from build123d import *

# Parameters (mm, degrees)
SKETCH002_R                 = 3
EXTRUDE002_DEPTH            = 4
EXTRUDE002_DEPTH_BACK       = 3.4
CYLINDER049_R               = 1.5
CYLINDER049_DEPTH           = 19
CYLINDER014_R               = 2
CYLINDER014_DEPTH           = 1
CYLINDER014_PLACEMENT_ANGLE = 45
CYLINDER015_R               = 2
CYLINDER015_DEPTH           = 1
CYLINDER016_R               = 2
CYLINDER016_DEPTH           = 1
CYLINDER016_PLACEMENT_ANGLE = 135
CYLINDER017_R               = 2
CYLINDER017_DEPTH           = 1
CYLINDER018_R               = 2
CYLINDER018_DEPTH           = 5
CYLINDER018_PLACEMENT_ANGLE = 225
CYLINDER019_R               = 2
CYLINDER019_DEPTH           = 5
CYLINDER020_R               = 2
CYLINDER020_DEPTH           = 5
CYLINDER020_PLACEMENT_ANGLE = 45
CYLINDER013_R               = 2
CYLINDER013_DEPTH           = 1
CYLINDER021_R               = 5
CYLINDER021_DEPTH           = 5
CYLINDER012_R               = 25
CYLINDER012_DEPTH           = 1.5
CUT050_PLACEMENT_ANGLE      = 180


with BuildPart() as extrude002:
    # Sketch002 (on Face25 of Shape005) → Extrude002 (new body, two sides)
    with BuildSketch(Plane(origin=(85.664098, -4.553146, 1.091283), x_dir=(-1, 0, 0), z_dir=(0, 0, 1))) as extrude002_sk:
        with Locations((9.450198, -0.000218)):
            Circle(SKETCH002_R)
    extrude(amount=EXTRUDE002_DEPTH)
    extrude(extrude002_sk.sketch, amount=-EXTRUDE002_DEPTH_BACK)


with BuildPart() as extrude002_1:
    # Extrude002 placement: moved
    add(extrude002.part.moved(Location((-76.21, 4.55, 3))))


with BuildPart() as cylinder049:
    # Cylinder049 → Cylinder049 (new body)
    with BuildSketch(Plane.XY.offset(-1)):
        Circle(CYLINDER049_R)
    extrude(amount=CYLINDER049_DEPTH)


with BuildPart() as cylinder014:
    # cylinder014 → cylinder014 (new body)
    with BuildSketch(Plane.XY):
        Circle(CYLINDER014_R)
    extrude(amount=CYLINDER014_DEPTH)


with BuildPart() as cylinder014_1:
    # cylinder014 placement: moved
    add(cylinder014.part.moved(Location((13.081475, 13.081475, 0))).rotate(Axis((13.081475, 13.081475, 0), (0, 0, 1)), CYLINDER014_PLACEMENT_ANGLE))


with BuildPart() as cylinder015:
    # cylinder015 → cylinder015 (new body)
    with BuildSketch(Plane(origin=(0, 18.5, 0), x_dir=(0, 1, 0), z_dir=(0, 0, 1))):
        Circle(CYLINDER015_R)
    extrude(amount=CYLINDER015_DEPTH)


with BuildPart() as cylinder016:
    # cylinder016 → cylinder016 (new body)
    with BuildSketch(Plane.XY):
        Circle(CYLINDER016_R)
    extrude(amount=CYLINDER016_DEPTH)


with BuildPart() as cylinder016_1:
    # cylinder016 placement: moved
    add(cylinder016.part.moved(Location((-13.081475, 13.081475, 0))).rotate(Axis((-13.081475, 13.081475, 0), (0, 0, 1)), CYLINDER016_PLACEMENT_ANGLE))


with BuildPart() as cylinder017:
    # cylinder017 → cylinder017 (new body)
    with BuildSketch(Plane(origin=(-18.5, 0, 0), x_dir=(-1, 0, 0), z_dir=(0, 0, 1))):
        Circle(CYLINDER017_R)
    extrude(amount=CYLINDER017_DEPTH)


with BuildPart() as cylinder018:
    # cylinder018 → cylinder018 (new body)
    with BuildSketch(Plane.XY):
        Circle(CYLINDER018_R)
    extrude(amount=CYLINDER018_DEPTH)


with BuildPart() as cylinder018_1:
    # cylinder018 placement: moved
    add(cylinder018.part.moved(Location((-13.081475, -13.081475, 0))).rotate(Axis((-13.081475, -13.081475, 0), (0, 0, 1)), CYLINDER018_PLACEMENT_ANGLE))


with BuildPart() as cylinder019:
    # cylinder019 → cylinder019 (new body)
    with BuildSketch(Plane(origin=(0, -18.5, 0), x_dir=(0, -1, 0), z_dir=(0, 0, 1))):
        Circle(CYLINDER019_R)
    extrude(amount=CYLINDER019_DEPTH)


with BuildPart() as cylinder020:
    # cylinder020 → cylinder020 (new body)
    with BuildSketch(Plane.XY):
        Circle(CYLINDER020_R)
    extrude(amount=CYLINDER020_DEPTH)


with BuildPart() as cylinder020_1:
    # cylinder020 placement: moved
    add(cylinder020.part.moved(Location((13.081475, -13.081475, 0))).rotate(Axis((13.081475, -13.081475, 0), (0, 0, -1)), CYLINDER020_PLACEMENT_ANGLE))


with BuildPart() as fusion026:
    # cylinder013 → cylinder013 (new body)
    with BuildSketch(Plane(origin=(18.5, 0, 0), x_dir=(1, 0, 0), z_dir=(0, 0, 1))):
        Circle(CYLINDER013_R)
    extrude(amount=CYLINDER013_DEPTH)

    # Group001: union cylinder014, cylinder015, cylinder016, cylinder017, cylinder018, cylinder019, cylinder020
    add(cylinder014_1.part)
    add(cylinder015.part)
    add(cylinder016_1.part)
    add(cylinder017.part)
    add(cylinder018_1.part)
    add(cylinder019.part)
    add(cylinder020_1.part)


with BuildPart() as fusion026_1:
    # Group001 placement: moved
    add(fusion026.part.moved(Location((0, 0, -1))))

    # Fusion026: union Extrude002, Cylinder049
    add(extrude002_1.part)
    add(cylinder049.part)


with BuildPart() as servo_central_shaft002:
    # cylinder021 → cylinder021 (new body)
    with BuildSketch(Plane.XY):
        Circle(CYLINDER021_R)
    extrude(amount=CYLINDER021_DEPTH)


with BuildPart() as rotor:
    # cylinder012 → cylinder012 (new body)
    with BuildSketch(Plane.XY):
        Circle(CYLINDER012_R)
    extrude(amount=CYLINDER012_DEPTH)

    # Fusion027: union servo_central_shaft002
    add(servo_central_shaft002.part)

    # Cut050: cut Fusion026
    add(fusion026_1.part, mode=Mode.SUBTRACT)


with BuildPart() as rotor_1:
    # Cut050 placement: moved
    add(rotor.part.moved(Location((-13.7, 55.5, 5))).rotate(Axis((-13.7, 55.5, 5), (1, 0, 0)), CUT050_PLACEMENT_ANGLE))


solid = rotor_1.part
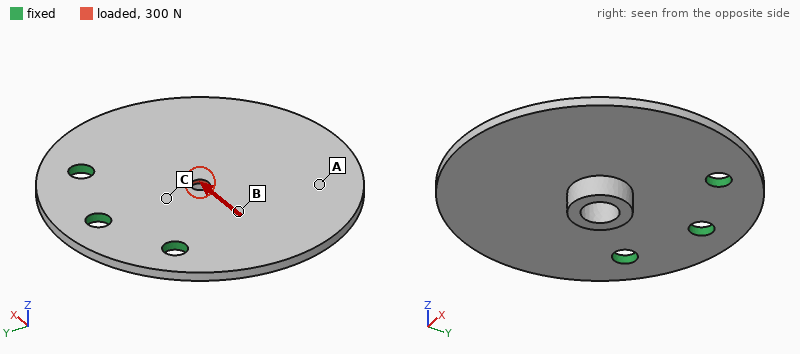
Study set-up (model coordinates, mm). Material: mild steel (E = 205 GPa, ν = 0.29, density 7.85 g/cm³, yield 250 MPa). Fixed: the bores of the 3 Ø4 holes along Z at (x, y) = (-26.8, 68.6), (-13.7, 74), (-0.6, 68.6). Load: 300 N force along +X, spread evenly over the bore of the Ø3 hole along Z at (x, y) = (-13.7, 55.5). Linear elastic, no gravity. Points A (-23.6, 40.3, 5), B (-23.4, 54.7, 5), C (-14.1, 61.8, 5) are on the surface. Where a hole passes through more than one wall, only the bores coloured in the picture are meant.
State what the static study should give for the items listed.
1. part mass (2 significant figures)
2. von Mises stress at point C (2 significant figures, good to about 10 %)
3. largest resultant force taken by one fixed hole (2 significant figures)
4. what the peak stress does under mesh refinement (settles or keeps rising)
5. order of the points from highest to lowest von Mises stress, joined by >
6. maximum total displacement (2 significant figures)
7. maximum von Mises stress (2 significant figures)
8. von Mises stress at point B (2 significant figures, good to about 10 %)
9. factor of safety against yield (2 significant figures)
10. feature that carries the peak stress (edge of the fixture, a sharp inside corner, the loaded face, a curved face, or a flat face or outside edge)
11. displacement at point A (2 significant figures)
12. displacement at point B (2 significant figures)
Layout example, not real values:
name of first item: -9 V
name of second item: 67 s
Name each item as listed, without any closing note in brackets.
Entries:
part mass: 24 g
von Mises stress at point C: 15 MPa
largest resultant force taken by one fixed hole: 190 N
what the peak stress does under mesh refinement: settles
order of the points from highest to lowest von Mises stress, joined by >: C > B > A
maximum total displacement: 3.4 µm
maximum von Mises stress: 81 MPa
von Mises stress at point B: 8.1 MPa
factor of safety against yield: 3.1
feature that carries the peak stress: the loaded face
displacement at point A: 2.4 µm
displacement at point B: 1.7 µm
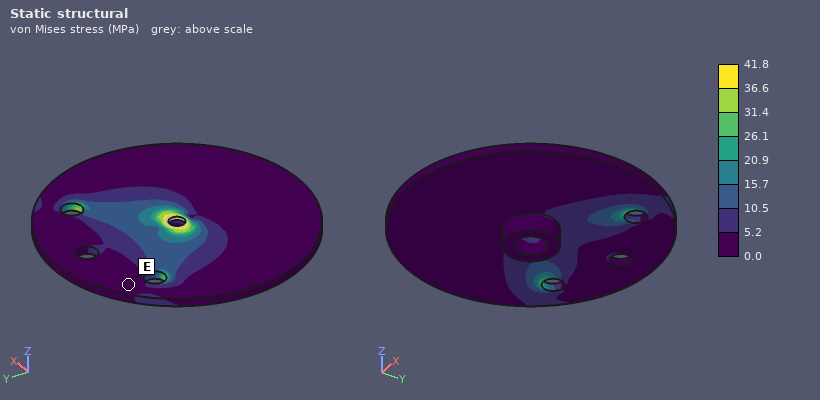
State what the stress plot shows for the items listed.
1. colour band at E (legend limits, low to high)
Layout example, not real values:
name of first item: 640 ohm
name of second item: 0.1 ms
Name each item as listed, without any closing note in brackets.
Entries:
colour band at E: 0.0 to 5.2 MPa
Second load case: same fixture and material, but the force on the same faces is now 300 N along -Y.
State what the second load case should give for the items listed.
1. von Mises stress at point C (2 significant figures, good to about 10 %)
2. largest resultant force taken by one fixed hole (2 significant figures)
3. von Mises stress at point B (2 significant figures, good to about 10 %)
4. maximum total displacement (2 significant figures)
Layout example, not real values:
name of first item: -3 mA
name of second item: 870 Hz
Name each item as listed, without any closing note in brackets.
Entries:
von Mises stress at point C: 20 MPa
largest resultant force taken by one fixed hole: 110 N
von Mises stress at point B: 5.4 MPa
maximum total displacement: 16 µm
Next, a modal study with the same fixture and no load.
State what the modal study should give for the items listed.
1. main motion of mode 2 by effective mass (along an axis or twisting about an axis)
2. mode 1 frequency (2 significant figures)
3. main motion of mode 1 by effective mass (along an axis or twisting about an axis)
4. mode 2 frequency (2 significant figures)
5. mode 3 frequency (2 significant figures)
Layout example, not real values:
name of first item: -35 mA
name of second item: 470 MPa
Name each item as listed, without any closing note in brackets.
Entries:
main motion of mode 2 by effective mass: twisting about Y
mode 1 frequency: 1100 Hz
main motion of mode 1 by effective mass: along Z
mode 2 frequency: 2600 Hz
mode 3 frequency: 4900 Hz
